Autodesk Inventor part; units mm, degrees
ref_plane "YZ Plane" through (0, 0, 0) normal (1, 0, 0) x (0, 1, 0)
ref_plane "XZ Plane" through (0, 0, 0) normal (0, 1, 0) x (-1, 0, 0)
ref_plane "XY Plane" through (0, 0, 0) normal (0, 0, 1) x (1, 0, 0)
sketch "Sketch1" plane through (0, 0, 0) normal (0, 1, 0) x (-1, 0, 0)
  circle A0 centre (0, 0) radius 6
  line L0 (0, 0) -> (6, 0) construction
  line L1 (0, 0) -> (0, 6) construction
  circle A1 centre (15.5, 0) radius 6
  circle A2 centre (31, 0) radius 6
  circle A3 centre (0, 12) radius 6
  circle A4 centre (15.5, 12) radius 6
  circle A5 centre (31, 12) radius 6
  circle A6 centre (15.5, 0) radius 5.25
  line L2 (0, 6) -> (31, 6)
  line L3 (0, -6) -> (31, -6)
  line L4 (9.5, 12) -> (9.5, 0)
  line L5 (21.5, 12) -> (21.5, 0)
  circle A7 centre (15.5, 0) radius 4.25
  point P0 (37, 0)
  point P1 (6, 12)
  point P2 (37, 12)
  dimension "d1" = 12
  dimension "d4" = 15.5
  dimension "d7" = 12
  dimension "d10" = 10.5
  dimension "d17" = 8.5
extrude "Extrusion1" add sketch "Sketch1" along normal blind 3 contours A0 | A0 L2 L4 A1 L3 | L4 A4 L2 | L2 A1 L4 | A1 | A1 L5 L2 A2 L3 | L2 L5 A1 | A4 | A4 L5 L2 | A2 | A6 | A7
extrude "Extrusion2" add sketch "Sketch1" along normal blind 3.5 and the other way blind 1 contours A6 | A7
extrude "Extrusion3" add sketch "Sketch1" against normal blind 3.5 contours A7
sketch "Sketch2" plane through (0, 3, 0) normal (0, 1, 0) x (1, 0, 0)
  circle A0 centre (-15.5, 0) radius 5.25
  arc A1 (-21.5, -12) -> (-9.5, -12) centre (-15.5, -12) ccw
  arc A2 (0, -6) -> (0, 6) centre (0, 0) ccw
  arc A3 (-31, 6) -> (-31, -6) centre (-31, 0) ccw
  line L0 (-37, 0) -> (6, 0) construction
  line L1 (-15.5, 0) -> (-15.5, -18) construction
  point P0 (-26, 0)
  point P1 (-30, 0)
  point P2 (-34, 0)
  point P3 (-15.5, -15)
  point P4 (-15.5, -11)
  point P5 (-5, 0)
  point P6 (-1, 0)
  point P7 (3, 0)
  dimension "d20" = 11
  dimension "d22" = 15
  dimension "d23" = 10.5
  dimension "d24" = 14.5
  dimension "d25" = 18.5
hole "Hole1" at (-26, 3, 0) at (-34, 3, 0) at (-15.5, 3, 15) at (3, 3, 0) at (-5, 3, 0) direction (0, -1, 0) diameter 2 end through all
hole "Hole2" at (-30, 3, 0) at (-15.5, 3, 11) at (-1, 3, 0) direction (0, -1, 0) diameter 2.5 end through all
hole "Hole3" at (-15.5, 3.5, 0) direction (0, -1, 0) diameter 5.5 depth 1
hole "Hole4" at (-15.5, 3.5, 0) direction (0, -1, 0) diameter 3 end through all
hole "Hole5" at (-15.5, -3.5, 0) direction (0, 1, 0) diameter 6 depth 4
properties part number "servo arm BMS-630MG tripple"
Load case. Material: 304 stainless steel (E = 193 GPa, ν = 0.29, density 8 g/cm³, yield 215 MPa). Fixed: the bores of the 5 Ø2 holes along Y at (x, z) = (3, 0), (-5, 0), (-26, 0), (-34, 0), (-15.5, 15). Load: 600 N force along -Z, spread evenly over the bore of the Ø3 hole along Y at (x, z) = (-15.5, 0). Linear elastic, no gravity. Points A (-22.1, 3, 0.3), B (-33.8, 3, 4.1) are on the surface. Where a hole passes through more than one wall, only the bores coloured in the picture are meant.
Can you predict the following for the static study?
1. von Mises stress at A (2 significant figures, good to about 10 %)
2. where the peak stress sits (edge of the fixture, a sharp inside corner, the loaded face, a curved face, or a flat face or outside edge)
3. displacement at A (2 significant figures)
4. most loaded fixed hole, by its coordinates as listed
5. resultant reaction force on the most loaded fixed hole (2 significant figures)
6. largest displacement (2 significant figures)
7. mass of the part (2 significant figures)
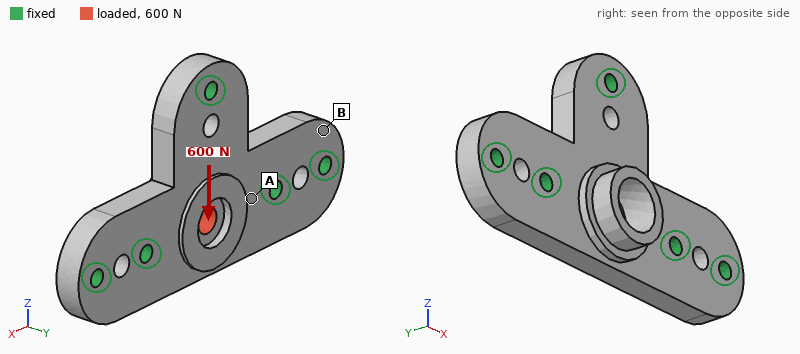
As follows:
10 MPa
the loaded face
0.47 µm
(-15.5, 15)
250 N
1.5 µm
15 g
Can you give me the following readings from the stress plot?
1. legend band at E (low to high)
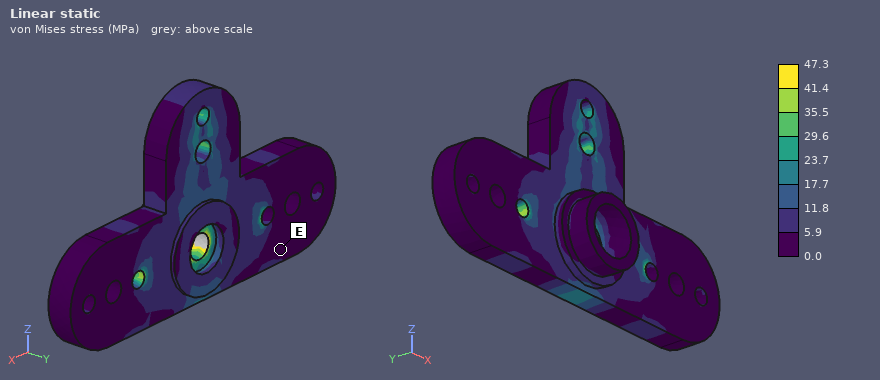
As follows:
0.0 to 5.9 MPa
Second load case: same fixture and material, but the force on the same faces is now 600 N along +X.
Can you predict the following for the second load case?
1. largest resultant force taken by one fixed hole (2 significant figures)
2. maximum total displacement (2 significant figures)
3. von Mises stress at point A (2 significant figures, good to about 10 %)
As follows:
240 N
0.82 µm
16 MPa
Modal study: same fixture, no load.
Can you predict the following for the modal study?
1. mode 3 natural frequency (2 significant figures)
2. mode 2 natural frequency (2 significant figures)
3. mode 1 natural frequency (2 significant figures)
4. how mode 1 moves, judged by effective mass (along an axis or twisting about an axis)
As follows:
51 kHz
35 kHz
28 kHz
along Y
